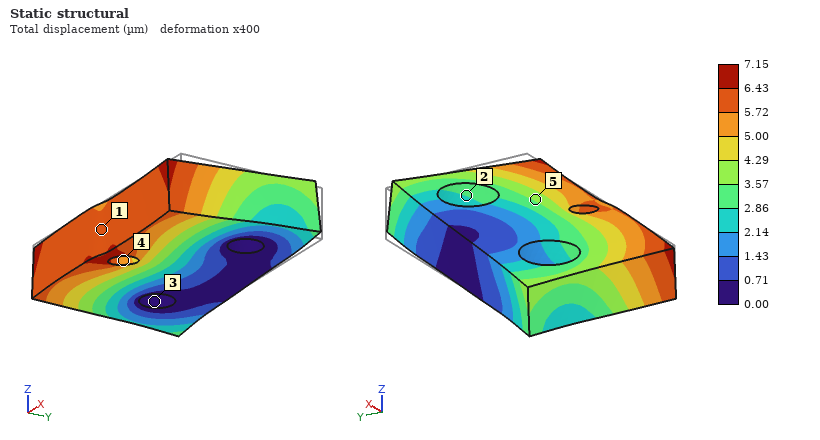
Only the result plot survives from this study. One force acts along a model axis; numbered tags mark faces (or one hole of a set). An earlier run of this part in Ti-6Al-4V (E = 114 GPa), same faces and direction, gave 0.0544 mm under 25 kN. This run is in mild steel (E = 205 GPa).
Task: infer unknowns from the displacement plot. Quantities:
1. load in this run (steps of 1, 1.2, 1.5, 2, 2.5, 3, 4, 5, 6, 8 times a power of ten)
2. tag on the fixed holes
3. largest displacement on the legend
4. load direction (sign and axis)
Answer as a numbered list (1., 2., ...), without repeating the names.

1. 6 kN
2. 3
3. 7.15 µm
4. -X
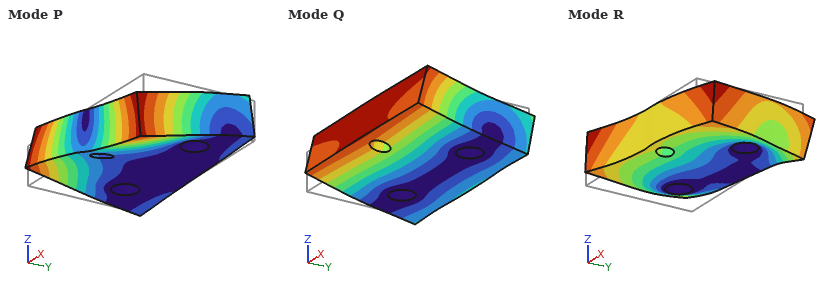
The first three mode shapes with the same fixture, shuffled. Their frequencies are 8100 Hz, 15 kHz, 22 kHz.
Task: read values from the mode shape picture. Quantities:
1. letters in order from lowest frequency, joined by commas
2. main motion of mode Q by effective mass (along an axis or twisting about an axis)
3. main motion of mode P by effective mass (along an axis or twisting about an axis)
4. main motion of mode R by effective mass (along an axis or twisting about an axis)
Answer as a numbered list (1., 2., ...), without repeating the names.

1. Q, P, R
2. along Z
3. twisting about Y
4. along X
